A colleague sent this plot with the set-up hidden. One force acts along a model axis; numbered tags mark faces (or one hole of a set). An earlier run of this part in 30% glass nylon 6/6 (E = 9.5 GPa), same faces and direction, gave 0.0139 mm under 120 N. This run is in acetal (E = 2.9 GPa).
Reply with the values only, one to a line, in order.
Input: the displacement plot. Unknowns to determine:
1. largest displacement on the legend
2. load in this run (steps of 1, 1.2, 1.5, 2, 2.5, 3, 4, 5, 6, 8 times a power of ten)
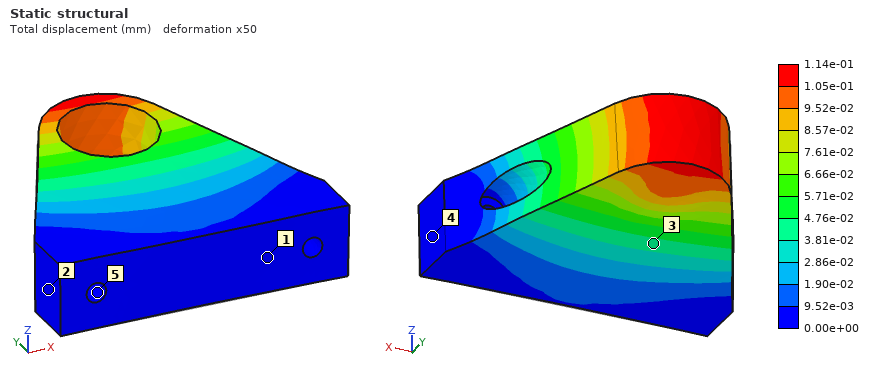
1.14e-01 mm
300 N
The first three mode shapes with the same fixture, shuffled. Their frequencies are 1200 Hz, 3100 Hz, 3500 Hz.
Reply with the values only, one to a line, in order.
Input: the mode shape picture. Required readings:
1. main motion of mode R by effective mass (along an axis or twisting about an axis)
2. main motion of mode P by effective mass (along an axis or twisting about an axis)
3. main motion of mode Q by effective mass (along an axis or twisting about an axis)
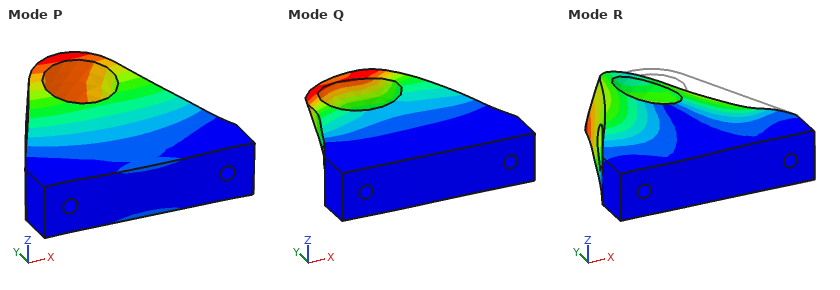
along X
along Z
along X
